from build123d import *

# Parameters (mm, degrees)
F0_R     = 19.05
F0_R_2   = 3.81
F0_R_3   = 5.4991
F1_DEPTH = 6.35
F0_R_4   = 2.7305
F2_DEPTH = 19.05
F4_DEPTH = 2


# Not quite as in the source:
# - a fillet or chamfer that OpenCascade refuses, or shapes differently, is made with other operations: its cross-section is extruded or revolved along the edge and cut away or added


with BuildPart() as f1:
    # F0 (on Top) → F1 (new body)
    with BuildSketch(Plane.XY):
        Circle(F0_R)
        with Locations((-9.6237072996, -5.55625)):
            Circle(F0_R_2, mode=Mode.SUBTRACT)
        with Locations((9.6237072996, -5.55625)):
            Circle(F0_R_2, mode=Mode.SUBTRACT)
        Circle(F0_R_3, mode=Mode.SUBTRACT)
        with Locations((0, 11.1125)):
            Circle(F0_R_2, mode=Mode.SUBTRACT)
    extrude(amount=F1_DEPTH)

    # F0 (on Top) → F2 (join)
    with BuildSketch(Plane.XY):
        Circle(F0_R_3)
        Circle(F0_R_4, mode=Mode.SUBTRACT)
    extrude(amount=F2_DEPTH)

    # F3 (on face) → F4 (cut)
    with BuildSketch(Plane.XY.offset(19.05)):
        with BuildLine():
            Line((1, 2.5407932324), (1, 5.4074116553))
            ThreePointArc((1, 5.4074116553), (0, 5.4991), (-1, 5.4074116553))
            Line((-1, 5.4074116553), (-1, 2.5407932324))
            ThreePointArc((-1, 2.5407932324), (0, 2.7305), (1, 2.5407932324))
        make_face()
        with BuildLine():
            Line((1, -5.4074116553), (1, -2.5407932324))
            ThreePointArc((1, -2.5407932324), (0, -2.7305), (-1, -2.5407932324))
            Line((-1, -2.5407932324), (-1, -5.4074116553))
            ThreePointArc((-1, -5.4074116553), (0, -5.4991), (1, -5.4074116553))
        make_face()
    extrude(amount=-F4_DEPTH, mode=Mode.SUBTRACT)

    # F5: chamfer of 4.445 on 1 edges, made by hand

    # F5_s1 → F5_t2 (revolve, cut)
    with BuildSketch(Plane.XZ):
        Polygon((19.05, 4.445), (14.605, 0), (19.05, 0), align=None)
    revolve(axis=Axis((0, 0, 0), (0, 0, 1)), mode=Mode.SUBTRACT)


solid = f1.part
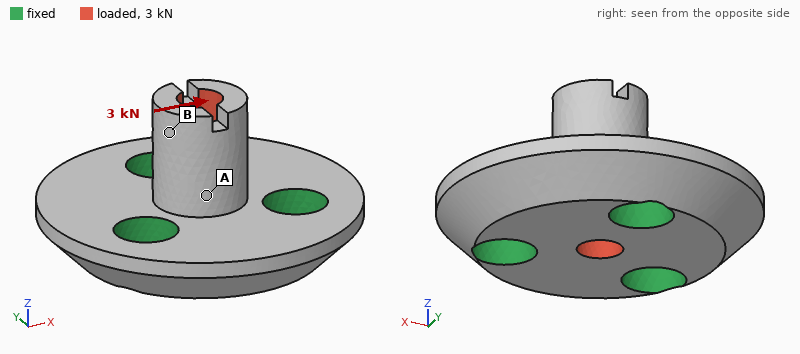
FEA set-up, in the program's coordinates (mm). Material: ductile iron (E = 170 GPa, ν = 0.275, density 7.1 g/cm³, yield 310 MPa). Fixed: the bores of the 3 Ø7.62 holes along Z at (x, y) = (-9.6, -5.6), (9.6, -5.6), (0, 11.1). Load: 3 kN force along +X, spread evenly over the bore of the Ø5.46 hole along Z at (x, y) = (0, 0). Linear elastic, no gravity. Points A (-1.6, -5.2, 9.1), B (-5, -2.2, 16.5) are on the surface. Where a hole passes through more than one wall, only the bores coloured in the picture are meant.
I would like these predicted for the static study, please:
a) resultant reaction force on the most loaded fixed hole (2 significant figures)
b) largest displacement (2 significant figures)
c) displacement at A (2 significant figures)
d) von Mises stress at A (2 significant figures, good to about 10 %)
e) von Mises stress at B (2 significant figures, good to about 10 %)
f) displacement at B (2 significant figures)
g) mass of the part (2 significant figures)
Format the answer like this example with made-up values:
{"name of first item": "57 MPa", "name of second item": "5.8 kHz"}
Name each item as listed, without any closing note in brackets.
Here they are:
{"resultant reaction force on the most loaded fixed hole": "1.5 kN", "largest displacement": "14 µm", "displacement at A": "3.6 µm", "von Mises stress at A": "47 MPa", "von Mises stress at B": "14 MPa", "displacement at B": "12 µm", "mass of the part": "43 g"}
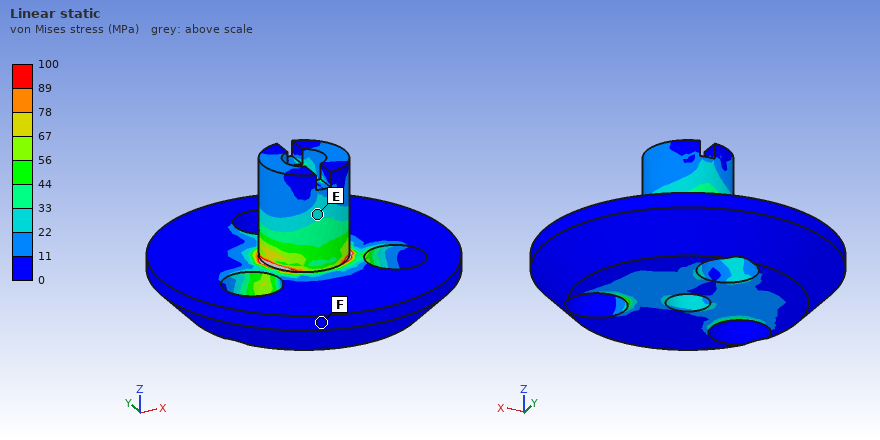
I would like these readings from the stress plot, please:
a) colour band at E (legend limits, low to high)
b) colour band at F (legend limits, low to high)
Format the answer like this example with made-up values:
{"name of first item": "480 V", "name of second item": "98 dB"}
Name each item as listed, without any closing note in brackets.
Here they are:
{"colour band at E": "22 to 33 MPa", "colour band at F": "0 to 11 MPa"}
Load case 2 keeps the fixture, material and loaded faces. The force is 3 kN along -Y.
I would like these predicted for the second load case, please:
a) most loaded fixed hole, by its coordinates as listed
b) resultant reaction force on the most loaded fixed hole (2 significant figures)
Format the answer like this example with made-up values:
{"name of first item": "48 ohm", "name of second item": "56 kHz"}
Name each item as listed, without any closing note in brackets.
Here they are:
{"most loaded fixed hole, by its coordinates as listed": "(0, 11.1)", "resultant reaction force on the most loaded fixed hole": "1.7 kN"}
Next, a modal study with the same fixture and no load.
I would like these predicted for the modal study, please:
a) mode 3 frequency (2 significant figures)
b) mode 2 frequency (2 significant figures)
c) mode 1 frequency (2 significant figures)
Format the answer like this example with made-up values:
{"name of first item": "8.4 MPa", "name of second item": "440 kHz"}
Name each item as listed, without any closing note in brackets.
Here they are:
{"mode 3 frequency": "43 kHz", "mode 2 frequency": "28 kHz", "mode 1 frequency": "28 kHz"}
